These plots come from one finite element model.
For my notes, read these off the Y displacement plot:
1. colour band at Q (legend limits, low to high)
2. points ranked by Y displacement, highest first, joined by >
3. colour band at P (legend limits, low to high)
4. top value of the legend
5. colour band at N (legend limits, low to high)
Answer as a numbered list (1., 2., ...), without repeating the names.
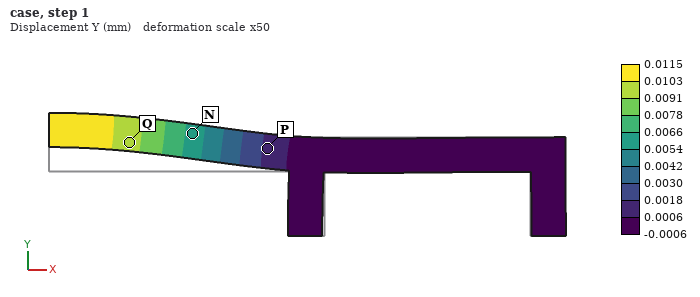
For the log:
1. 0.0091 to 0.0103 mm
2. Q > N > P
3. 0.0006 to 0.0018 mm
4. 0.0115 mm
5. 0.0054 to 0.0066 mm
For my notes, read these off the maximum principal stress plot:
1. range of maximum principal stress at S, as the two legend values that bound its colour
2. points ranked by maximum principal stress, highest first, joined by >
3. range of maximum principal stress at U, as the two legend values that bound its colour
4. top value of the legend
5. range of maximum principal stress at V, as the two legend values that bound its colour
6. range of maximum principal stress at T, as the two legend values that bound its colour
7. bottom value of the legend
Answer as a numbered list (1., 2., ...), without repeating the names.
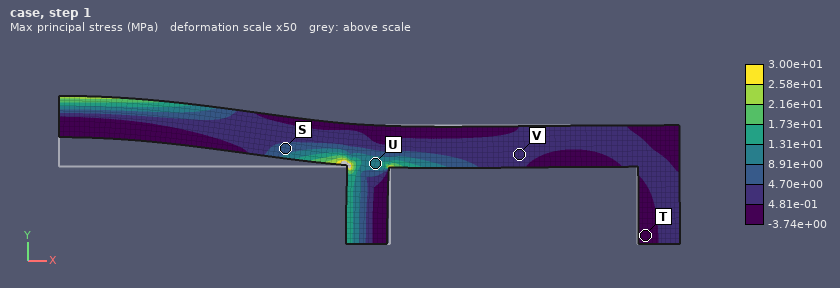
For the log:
1. 4.70e+00 to 8.91e+00 MPa
2. U > S > V > T
3. 8.91e+00 to 1.31e+01 MPa
4. 3.00e+01 MPa
5. 4.81e-01 to 4.70e+00 MPa
6. -3.74e+00 to 4.81e-01 MPa
7. -3.74e+00 MPa
